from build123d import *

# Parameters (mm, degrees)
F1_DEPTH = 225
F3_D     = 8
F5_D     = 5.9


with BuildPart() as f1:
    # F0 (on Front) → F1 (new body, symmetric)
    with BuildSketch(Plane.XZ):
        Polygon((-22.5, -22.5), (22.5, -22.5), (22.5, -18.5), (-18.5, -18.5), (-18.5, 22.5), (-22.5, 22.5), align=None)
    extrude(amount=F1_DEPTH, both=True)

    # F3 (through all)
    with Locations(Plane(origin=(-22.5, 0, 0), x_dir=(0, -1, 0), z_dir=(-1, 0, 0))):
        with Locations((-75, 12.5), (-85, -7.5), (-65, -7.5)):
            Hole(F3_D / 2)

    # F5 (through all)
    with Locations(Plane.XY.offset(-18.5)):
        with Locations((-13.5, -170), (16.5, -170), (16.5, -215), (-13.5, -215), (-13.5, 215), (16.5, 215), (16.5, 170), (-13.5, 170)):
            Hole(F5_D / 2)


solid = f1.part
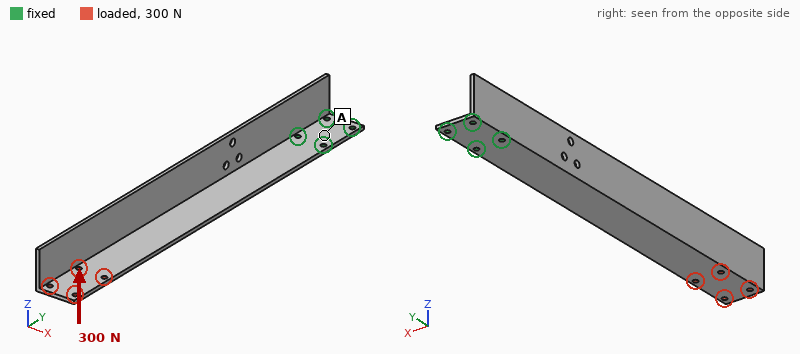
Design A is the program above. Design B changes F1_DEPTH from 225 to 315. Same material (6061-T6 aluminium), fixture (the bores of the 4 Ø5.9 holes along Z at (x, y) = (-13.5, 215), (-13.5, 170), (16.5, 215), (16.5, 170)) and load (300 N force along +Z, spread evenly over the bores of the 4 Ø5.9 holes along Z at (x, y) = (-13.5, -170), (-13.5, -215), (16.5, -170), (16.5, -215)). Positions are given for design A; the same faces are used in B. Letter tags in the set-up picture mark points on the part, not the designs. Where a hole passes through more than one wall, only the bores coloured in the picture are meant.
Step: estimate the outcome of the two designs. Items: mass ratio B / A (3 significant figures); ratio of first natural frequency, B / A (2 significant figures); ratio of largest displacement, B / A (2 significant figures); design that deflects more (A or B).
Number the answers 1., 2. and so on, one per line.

1. 1.40
2. 0.68
3. 1.1
4. B
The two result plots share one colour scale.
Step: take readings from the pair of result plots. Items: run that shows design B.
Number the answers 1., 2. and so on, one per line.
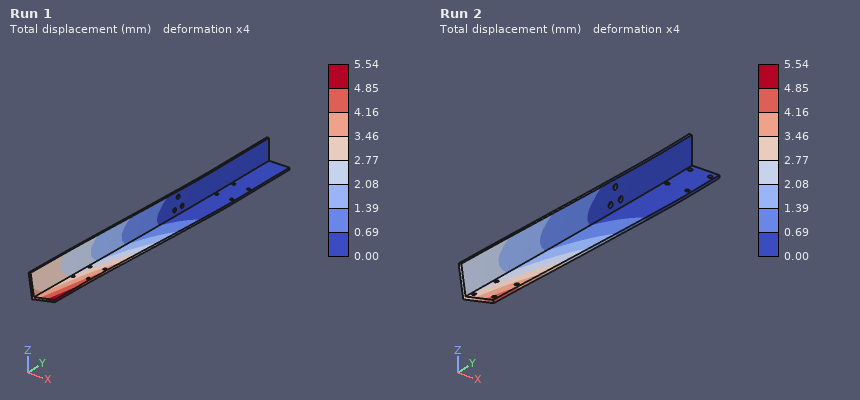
1. Run 1
